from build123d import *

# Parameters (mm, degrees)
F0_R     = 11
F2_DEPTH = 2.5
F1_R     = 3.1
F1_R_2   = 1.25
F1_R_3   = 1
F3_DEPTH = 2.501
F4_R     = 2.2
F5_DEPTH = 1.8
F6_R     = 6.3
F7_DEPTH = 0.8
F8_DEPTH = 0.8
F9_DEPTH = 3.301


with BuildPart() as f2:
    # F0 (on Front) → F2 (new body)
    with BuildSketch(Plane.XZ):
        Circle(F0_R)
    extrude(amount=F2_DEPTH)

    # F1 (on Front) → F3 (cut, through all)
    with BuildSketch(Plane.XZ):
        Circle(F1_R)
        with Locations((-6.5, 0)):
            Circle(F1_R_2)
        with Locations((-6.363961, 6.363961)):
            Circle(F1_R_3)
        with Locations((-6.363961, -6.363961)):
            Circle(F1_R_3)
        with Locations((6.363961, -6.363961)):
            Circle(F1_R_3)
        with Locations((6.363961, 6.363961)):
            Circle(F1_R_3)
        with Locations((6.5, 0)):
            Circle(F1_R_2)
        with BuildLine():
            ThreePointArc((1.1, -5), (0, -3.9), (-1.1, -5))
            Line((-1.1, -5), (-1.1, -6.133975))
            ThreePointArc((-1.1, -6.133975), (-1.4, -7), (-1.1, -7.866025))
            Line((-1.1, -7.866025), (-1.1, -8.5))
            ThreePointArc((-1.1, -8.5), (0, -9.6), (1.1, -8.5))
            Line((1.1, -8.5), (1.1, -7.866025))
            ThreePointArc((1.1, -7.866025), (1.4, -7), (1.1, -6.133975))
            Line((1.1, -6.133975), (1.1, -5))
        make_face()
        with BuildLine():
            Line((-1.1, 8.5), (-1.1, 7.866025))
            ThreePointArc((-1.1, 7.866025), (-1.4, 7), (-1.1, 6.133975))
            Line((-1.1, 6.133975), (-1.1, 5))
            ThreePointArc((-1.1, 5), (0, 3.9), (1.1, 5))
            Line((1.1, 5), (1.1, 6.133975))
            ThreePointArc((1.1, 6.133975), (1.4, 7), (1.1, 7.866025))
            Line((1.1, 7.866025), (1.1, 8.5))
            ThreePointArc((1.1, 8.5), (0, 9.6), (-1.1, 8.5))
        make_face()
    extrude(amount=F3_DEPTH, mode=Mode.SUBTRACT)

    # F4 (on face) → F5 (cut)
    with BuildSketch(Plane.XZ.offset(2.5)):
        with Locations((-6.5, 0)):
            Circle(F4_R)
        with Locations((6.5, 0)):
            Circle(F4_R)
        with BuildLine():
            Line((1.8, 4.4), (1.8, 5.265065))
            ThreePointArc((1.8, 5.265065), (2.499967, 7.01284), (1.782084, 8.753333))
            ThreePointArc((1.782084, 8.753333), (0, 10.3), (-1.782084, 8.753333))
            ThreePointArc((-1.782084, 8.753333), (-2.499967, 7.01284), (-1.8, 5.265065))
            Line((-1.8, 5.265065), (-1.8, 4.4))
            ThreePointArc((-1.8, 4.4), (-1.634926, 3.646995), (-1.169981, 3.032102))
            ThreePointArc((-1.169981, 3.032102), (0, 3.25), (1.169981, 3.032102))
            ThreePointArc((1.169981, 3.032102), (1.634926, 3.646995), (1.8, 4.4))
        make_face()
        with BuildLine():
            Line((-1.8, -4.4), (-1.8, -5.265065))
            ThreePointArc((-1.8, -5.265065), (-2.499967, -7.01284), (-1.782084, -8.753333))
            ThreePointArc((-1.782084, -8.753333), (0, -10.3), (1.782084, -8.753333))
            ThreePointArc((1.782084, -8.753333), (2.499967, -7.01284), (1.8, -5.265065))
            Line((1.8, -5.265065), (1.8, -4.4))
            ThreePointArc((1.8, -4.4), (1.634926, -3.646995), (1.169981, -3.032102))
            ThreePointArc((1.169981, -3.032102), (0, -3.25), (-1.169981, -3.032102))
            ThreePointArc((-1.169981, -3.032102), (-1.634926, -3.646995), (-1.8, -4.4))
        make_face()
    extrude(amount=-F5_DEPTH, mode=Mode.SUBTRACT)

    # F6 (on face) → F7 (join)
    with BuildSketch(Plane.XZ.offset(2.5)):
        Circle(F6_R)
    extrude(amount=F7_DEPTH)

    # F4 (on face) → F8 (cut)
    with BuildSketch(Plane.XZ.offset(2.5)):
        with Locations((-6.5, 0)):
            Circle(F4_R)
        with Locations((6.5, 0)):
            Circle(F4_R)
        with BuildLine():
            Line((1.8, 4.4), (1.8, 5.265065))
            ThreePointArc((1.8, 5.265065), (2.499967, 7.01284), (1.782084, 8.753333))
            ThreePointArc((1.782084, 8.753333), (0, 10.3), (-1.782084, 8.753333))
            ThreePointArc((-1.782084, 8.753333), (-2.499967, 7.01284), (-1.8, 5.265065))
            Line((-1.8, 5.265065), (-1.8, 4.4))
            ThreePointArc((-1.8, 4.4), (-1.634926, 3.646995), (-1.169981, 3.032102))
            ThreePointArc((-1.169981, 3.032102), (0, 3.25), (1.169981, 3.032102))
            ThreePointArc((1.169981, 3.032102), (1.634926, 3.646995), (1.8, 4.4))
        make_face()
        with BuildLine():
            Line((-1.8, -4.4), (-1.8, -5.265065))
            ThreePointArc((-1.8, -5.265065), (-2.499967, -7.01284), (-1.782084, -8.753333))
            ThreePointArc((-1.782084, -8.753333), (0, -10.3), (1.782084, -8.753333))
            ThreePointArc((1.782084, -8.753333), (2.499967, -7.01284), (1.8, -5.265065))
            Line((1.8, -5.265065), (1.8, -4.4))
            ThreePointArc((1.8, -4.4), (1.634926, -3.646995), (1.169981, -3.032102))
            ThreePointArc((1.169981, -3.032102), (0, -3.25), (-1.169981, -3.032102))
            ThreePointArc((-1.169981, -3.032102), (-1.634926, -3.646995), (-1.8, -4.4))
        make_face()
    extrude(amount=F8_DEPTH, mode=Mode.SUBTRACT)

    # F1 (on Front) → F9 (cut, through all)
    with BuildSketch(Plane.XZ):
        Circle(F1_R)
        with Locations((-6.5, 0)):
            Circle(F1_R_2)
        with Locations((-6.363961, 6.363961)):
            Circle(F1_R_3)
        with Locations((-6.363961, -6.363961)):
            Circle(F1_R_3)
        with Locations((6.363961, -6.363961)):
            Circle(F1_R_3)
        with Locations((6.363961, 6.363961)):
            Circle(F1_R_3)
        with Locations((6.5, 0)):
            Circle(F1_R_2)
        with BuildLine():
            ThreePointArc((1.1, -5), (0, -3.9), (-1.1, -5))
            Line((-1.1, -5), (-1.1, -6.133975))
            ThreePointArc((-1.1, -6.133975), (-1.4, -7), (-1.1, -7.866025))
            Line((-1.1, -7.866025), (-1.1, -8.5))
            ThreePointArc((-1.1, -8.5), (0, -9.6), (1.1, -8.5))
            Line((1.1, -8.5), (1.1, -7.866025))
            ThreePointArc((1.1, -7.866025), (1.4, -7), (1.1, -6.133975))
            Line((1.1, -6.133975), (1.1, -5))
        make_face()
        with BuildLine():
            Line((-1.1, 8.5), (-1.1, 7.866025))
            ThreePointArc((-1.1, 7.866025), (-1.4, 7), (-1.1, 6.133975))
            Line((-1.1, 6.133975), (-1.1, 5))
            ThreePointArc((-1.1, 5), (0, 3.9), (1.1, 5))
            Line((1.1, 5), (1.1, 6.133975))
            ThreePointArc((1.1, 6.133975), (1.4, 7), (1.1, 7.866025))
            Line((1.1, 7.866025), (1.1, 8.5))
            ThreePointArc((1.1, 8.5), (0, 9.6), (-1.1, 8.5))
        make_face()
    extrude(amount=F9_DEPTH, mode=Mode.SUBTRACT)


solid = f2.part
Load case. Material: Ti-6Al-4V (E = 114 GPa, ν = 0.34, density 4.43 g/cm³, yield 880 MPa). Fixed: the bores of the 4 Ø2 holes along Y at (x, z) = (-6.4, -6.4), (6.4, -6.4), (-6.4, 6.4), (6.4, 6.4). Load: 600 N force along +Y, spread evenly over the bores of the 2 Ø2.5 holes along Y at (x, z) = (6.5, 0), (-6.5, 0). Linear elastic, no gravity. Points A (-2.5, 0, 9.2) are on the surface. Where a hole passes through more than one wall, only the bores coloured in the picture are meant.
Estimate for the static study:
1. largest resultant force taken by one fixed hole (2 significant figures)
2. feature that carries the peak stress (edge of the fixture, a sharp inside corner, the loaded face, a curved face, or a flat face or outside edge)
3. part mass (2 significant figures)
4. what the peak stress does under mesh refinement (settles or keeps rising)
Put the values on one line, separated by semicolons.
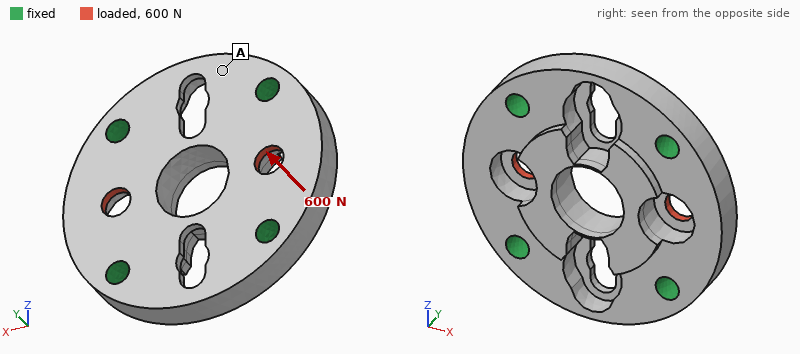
150 N; a sharp inside corner; 3.2 g; keeps rising
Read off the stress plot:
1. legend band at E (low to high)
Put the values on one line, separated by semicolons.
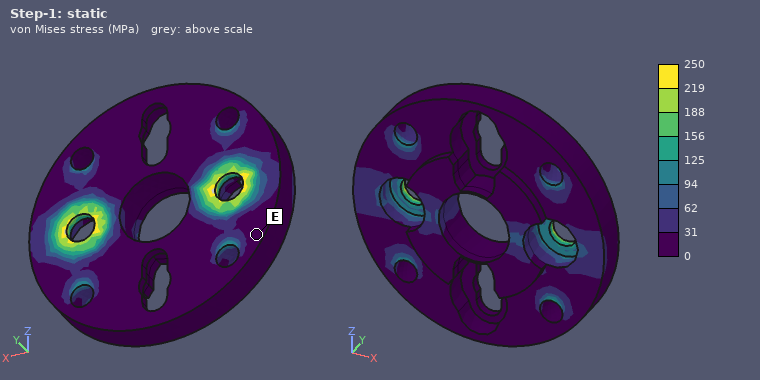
0 to 31 MPa
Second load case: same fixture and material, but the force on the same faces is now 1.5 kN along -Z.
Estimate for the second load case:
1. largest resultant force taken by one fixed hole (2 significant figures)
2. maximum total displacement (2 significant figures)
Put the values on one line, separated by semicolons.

380 N; 3.7 µm
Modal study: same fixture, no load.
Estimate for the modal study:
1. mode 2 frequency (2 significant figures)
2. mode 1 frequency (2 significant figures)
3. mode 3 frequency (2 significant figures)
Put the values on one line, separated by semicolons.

62 kHz; 59 kHz; 62 kHz
